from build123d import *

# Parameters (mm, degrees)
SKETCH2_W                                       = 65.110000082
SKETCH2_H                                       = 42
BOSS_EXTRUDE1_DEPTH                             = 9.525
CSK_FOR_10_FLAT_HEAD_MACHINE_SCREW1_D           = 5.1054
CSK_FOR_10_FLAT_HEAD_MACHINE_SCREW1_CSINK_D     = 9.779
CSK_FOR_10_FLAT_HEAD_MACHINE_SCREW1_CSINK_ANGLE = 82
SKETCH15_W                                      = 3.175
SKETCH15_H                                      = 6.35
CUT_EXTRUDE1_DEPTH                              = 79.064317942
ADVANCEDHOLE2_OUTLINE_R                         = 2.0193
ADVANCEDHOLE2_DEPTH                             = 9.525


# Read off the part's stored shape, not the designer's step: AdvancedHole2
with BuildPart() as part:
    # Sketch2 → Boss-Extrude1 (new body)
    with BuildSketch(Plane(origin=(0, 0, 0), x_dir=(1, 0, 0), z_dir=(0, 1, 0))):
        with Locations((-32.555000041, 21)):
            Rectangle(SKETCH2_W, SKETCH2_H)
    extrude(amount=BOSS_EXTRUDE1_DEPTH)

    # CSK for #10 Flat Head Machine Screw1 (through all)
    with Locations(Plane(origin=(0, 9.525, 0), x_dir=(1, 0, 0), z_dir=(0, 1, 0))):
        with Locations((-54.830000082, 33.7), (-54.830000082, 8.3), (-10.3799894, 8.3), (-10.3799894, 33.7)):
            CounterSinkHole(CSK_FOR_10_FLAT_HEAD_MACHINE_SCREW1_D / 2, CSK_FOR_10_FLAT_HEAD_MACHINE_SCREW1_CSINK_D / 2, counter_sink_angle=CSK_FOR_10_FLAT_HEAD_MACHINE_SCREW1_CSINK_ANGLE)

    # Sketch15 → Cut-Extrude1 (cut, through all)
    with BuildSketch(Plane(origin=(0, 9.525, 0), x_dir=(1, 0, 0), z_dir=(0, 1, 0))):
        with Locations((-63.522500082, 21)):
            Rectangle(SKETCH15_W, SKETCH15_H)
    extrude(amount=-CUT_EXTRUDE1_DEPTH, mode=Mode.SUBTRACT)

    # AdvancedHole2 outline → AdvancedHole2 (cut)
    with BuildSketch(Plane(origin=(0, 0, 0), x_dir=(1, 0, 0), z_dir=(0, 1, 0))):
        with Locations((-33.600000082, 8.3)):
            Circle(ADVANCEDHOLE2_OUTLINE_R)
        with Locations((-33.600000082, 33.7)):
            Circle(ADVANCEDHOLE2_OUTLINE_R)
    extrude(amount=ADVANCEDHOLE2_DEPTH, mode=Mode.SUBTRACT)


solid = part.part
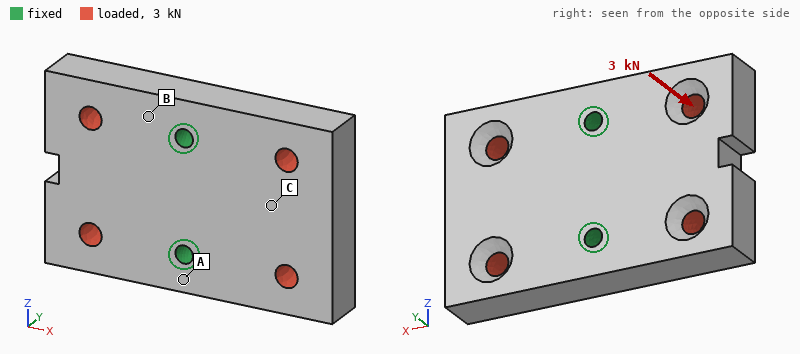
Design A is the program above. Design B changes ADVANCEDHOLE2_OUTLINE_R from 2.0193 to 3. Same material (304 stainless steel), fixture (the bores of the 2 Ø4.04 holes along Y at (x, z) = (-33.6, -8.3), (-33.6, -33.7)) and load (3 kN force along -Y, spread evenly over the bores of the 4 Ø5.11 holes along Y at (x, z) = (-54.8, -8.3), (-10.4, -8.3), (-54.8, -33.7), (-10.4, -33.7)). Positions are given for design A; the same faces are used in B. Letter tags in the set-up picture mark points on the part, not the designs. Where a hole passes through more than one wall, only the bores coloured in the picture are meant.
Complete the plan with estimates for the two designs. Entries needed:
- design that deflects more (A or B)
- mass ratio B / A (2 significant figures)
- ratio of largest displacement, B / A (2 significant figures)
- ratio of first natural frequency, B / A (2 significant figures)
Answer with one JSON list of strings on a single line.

["A", "0.99", "0.91", "1.1"]
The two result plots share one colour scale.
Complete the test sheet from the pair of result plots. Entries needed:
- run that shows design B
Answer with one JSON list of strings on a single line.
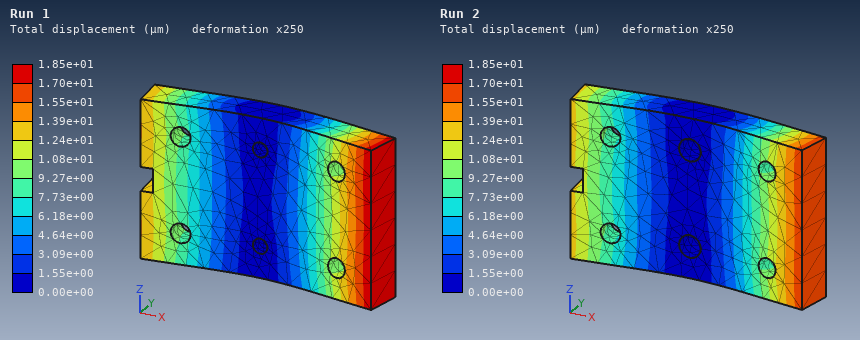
["Run 2"]
